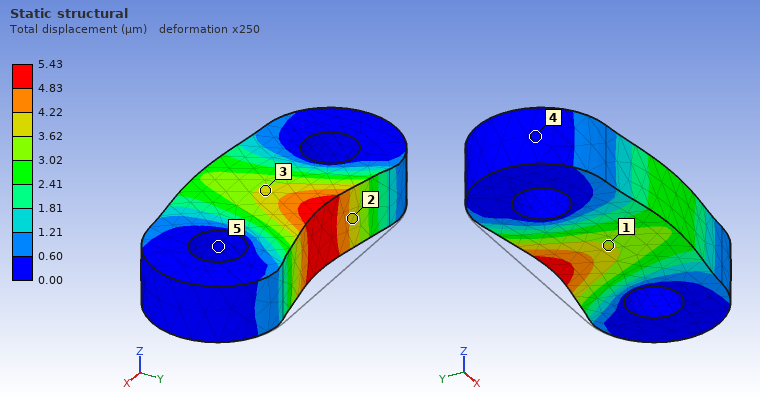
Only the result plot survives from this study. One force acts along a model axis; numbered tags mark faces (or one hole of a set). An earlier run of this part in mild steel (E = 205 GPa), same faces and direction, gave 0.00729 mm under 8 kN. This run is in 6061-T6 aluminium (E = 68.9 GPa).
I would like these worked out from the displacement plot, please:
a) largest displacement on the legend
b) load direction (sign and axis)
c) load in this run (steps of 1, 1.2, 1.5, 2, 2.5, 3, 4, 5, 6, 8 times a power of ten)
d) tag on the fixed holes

5.43 µm
-Y
2 kN
5
